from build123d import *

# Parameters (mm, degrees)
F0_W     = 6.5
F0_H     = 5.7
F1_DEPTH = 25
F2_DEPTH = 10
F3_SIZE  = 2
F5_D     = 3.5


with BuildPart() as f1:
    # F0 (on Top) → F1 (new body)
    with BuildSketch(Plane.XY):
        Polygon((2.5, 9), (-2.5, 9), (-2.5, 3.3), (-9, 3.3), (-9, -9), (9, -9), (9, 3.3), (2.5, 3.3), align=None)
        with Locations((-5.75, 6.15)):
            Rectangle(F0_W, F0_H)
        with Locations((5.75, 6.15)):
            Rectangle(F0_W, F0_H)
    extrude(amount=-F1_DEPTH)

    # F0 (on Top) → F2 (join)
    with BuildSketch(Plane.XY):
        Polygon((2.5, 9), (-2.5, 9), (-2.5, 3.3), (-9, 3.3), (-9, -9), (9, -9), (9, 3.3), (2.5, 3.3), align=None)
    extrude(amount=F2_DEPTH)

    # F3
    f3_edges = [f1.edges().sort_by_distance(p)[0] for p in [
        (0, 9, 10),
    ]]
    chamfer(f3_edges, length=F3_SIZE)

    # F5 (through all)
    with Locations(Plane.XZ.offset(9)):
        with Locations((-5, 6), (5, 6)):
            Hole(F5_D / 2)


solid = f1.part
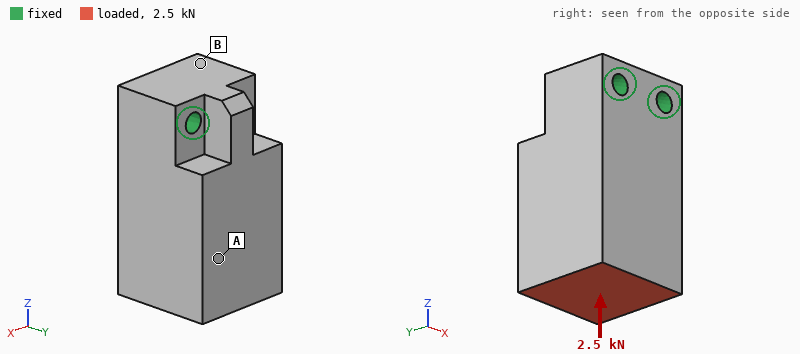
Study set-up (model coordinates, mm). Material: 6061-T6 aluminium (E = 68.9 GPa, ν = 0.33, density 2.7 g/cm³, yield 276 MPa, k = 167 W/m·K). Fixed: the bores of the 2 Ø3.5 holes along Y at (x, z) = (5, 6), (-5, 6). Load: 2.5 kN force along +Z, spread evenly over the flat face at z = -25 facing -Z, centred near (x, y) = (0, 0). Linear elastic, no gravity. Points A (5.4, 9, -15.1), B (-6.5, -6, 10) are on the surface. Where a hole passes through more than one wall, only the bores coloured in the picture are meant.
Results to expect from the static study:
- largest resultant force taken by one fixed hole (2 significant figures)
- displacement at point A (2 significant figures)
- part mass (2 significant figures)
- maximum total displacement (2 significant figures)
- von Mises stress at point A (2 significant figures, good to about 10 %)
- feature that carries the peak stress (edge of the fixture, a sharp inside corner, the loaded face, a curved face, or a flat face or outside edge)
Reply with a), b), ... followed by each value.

a) 1.3 kN
b) 7.4 µm
c) 28 g
d) 9.8 µm
e) 7.6 MPa
f) edge of the fixture
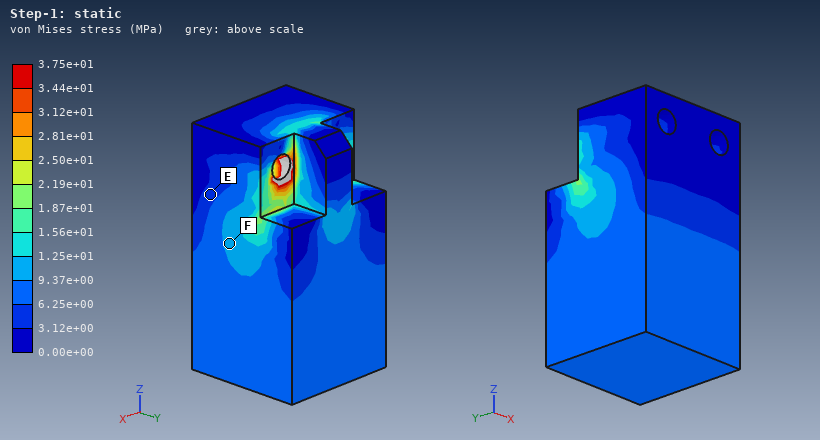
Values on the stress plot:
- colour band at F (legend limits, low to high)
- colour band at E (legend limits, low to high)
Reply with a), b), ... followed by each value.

a) 9.37e+00 to 1.25e+01 MPa
b) 3.12e+00 to 6.25e+00 MPa
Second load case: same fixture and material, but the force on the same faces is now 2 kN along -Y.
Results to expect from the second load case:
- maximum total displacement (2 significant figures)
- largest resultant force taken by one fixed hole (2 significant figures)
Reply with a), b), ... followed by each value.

a) 83 µm
b) 1.0 kN
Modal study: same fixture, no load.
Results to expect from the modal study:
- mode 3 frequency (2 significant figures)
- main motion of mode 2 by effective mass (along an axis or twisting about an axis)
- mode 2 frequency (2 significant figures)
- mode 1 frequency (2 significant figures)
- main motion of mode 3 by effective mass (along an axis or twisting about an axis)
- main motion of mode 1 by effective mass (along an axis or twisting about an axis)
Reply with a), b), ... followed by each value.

a) 20 kHz
b) along X
c) 11 kHz
d) 8800 Hz
e) twisting about Z
f) along Y
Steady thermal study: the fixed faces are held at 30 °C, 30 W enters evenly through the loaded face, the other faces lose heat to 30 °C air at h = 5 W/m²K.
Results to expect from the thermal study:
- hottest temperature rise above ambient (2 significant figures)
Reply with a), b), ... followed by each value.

a) 18 K
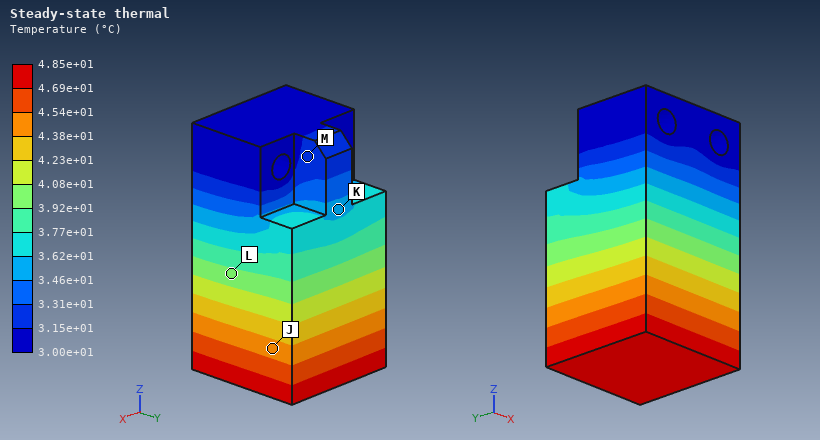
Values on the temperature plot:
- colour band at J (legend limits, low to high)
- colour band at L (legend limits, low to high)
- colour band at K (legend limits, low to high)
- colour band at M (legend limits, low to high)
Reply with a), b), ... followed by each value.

a) 4.38e+01 to 4.54e+01 °C
b) 3.92e+01 to 4.08e+01 °C
c) 3.46e+01 to 3.62e+01 °C
d) 3.15e+01 to 3.31e+01 °C
